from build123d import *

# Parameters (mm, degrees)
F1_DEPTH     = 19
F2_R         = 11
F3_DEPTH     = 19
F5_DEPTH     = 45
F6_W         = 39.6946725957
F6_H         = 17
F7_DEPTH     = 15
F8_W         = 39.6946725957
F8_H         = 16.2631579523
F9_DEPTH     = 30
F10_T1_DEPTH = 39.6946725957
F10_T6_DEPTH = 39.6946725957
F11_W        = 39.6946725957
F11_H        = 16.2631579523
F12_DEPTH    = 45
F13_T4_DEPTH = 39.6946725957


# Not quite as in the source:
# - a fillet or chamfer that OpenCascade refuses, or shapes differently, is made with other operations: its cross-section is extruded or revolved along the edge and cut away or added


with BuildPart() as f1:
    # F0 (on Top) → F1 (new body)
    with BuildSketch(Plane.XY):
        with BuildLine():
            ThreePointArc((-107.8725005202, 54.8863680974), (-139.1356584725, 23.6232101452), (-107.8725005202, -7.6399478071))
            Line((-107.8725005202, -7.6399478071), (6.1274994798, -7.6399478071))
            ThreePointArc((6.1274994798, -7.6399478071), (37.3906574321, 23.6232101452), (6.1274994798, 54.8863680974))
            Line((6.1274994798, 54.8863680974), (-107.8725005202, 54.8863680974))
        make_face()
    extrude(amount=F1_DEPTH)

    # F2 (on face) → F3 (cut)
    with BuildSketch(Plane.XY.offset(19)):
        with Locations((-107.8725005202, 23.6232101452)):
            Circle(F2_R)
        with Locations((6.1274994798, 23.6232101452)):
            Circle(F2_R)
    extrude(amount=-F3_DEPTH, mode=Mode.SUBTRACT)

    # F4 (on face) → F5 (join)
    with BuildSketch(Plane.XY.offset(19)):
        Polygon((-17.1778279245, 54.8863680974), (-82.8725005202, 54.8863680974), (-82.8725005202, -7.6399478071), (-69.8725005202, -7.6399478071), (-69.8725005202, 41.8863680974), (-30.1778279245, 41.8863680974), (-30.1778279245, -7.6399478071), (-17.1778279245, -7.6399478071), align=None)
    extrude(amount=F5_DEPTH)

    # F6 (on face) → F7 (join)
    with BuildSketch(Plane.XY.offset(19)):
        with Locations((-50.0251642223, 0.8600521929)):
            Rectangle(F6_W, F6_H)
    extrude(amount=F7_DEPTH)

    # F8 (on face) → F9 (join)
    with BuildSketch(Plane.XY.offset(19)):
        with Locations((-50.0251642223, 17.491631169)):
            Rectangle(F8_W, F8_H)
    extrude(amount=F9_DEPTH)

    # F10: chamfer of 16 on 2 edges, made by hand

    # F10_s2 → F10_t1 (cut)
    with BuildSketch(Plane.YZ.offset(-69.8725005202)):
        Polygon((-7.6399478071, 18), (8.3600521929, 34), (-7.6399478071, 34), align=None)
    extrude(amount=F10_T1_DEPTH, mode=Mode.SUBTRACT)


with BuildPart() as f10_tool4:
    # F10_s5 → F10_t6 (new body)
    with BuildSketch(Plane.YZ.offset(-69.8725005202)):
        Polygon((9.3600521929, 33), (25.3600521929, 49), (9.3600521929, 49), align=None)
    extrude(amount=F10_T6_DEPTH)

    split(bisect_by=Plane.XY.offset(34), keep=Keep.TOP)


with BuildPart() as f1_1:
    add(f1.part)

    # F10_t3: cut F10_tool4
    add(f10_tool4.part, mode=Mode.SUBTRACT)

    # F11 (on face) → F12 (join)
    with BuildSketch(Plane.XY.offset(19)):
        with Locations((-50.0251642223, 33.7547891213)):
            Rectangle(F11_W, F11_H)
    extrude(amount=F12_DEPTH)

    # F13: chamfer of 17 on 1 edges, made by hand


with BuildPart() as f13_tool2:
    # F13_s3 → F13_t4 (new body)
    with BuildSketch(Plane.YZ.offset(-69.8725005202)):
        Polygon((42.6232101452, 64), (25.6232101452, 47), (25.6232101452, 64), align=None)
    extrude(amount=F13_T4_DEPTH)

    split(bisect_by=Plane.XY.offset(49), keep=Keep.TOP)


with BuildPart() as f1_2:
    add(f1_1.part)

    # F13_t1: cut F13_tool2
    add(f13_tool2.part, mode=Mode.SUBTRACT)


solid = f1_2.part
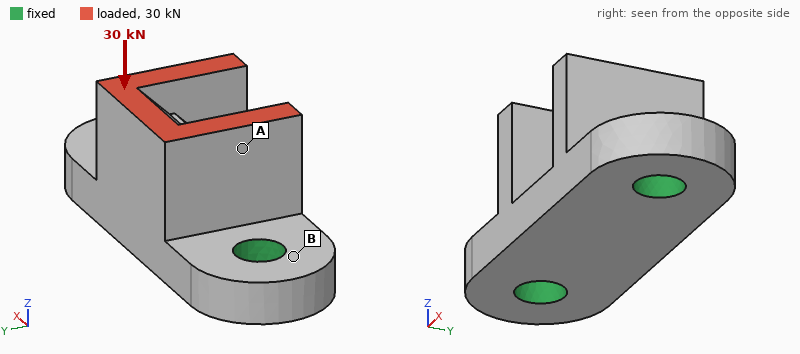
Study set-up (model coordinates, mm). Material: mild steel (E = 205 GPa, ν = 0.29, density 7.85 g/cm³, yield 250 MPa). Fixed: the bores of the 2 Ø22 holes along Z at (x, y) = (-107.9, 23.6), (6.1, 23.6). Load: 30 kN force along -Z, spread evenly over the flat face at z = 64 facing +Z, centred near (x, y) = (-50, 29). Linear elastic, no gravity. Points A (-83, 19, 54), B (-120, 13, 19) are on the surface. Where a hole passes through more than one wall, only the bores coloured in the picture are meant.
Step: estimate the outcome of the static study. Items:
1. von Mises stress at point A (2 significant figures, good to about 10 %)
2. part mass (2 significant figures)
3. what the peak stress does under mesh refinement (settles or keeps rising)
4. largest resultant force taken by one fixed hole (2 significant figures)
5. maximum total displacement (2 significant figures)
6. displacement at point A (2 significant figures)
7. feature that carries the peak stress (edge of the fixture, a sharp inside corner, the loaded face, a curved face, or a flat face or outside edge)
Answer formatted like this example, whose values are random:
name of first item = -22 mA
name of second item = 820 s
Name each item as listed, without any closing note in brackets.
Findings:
von Mises stress at point A = 16 MPa
part mass = 2.5 kg
what the peak stress does under mesh refinement = keeps rising
largest resultant force taken by one fixed hole = 16 kN
maximum total displacement = 21 µm
displacement at point A = 13 µm
feature that carries the peak stress = edge of the fixture
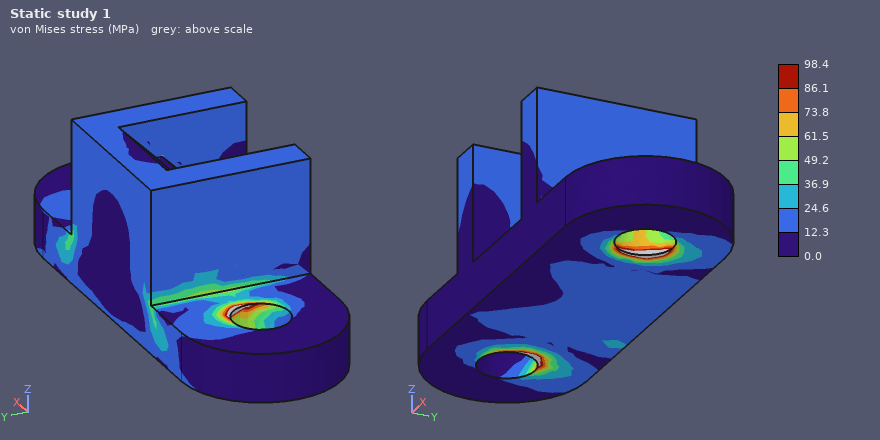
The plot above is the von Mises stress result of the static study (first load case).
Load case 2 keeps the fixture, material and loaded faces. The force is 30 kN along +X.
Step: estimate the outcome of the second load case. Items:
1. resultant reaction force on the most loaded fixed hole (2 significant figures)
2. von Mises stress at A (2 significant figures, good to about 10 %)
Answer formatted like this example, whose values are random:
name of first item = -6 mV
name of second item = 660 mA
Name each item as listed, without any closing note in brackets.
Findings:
resultant reaction force on the most loaded fixed hole = 25 kN
von Mises stress at A = 70 MPa
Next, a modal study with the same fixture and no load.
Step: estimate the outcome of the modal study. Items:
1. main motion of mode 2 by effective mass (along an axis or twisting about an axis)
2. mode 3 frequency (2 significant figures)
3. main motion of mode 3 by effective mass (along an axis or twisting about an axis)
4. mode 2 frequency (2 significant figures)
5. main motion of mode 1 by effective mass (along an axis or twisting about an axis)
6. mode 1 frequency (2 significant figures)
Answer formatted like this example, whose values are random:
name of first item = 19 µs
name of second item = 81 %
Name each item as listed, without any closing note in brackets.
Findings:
main motion of mode 2 by effective mass = along Z
mode 3 frequency = 7300 Hz
main motion of mode 3 by effective mass = along X
mode 2 frequency = 6500 Hz
main motion of mode 1 by effective mass = along Y
mode 1 frequency = 3600 Hz
